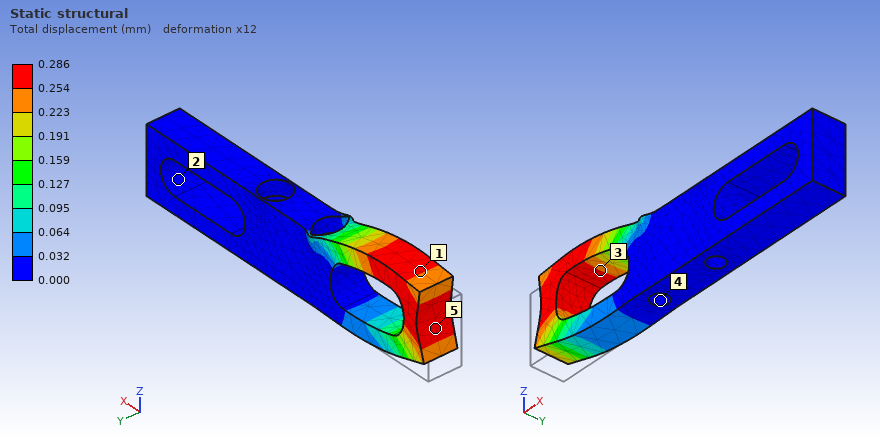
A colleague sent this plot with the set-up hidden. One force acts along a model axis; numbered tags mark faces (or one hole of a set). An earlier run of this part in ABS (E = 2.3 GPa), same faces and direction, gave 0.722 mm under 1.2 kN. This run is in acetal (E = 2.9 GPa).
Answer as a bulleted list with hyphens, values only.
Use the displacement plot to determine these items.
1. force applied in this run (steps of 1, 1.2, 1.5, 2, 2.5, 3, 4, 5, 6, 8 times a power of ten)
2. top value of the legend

- 600 N
- 0.286 mm
